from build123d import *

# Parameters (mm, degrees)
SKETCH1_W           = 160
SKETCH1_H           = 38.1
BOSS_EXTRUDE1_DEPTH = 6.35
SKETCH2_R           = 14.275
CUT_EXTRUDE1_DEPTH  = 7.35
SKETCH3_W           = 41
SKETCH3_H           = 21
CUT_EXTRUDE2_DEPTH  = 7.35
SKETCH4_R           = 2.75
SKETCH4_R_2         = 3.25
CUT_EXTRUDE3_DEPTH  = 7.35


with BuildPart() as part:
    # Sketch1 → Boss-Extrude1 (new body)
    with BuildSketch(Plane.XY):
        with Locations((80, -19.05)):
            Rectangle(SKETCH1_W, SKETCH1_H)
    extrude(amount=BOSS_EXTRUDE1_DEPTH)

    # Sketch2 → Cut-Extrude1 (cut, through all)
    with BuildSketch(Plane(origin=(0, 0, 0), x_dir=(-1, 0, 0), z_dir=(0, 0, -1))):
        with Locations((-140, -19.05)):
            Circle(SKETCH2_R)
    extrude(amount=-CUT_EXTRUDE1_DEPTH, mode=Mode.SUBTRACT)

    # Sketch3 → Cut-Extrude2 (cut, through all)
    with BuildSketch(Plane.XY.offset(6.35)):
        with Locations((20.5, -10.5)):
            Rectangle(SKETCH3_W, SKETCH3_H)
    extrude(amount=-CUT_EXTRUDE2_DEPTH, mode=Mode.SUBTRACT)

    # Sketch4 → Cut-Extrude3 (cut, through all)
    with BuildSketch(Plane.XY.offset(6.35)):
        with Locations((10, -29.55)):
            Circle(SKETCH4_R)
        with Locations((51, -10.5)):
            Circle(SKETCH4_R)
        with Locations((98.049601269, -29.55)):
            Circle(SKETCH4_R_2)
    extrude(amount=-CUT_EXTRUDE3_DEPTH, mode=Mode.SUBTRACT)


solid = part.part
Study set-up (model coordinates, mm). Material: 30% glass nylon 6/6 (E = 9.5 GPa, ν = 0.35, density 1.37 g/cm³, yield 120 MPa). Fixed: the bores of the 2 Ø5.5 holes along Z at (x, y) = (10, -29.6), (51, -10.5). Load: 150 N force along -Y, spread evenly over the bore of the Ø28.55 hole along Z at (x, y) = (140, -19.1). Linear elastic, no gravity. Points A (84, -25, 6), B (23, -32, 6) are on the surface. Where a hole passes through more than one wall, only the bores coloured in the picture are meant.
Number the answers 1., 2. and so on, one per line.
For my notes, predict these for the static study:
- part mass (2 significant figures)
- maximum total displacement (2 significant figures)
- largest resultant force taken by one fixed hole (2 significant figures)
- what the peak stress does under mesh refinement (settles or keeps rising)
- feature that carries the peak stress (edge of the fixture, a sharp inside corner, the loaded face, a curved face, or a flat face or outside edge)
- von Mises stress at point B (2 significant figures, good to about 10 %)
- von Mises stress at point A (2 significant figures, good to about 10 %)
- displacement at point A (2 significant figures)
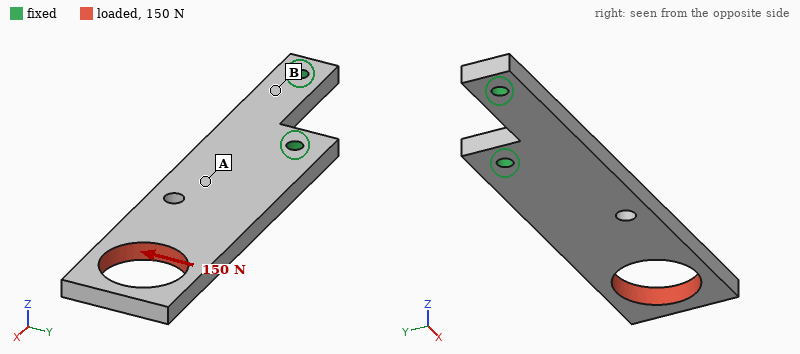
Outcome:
1. 39 g
2. 0.37 mm
3. 490 N
4. keeps rising
5. edge of the fixture
6. 5.1 MPa
7. 2.5 MPa
8. 0.068 mm
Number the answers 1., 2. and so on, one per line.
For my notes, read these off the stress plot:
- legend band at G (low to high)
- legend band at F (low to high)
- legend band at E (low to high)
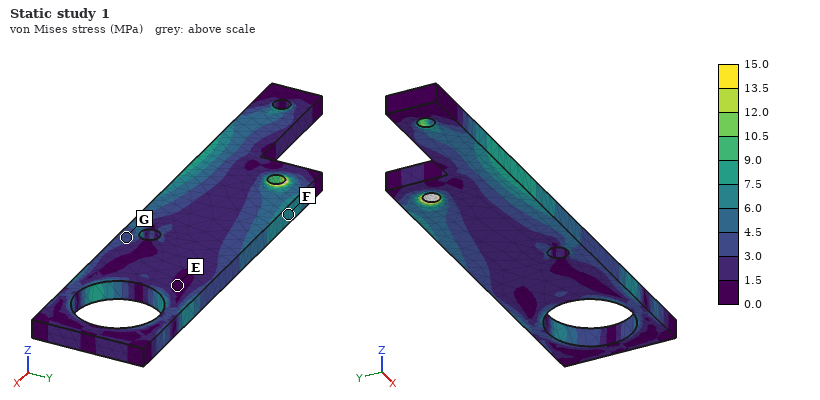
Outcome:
1. 3.0 to 4.5 MPa
2. 6.0 to 7.5 MPa
3. 0.0 to 1.5 MPa
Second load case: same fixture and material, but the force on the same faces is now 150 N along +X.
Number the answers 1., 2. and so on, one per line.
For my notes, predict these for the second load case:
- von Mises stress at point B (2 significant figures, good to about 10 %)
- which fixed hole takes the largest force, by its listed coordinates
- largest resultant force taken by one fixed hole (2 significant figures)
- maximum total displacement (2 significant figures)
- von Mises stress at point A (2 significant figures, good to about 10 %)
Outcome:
1. 0.56 MPa
2. (51, -10.5)
3. 99 N
4. 21 µm
5. 0.57 MPa
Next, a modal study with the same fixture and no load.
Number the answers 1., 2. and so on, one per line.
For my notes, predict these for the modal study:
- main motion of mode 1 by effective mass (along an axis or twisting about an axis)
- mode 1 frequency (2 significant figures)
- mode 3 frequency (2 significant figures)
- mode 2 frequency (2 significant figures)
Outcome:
1. along Z
2. 270 Hz
3. 1100 Hz
4. 1100 Hz
